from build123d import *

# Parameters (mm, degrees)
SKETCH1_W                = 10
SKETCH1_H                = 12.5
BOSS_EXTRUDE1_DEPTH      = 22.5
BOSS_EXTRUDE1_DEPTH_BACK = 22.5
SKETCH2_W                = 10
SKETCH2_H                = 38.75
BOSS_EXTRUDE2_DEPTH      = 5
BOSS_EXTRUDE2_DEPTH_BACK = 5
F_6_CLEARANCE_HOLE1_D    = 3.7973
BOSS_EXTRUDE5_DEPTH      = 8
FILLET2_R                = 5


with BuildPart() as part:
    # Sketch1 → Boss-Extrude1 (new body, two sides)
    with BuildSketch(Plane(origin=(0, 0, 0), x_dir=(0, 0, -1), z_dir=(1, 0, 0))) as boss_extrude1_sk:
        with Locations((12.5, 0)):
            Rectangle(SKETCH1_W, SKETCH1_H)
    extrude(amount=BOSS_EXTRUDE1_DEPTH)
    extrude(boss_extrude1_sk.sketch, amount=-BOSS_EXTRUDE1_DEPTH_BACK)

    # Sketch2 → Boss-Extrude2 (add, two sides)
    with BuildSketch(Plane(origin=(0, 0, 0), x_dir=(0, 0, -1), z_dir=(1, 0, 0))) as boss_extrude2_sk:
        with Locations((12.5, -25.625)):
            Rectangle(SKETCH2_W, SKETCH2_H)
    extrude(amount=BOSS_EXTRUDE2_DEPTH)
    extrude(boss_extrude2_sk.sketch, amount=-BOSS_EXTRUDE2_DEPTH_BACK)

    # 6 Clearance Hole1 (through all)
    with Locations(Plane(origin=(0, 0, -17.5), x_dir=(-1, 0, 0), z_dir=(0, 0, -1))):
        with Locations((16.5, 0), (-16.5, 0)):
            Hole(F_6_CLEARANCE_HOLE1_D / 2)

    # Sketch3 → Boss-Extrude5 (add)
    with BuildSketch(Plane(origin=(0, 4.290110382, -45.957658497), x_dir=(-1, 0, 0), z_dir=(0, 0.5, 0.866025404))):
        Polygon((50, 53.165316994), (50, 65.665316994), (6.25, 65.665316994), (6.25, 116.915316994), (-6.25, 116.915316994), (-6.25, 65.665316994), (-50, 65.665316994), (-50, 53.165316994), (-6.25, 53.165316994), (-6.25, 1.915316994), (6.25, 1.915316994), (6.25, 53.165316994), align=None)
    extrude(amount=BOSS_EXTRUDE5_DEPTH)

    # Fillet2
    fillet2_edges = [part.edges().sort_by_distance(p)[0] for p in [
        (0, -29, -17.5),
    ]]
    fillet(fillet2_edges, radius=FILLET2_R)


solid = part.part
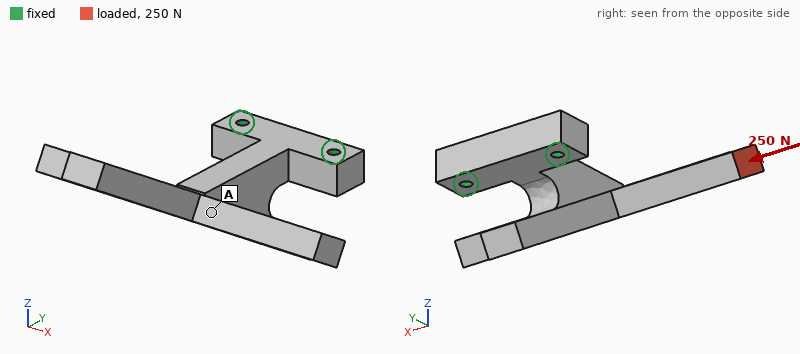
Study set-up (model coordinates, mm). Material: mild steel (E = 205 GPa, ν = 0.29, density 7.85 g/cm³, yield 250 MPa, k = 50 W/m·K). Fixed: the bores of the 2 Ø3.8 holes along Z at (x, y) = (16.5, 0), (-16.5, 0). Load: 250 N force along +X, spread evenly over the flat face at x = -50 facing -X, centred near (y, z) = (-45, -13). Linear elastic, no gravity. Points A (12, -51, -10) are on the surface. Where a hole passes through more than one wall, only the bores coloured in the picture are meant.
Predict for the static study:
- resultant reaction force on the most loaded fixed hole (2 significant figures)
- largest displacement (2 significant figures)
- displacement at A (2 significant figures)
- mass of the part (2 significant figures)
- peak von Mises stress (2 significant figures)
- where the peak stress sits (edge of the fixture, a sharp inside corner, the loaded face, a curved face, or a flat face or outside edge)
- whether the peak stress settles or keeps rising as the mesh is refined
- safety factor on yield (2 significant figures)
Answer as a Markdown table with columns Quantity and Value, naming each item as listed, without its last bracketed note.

| Quantity | Value |
|---|---|
| resultant reaction force on the most loaded fixed hole | 420 N |
| largest displacement | 91 µm |
| displacement at A | 42 µm |
| mass of the part | 230 g |
| peak von Mises stress | 65 MPa |
| where the peak stress sits | a curved face |
| whether the peak stress settles or keeps rising as the mesh is refined | settles |
| safety factor on yield | 3.8 |
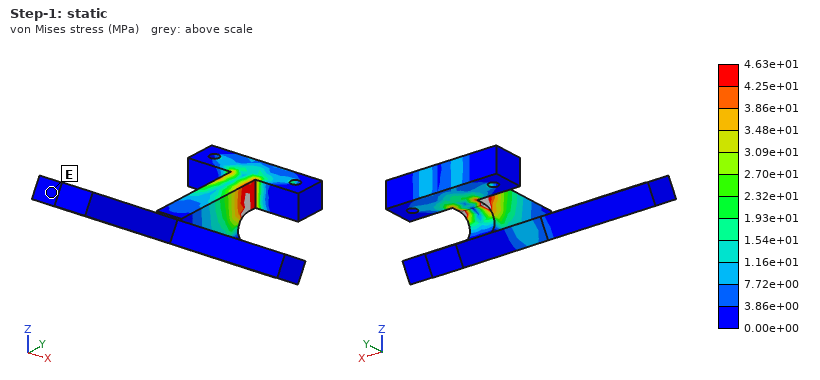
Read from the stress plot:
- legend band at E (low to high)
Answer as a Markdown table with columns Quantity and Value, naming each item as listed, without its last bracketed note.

| Quantity | Value |
|---|---|
| legend band at E | 0.00e+00 to 3.86e+00 MPa |
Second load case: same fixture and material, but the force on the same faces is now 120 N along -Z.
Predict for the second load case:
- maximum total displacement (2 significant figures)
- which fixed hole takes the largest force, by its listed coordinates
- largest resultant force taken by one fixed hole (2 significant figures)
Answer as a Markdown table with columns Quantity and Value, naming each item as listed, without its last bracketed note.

| Quantity | Value |
|---|---|
| maximum total displacement | 0.12 mm |
| which fixed hole takes the largest force, by its listed coordinates | (-16.5, 0) |
| largest resultant force taken by one fixed hole | 290 N |
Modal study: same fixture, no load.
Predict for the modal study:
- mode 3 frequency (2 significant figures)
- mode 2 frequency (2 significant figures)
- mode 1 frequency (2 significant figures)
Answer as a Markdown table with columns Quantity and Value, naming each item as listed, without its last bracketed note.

| Quantity | Value |
|---|---|
| mode 3 frequency | 1200 Hz |
| mode 2 frequency | 740 Hz |
| mode 1 frequency | 720 Hz |
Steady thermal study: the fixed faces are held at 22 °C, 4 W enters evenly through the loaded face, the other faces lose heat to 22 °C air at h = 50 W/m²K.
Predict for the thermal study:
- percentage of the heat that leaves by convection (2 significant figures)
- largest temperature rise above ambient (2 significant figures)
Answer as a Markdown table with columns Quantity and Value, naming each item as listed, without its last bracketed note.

| Quantity | Value |
|---|---|
| percentage of the heat that leaves by convection | 82 % |
| largest temperature rise above ambient | 33 K |
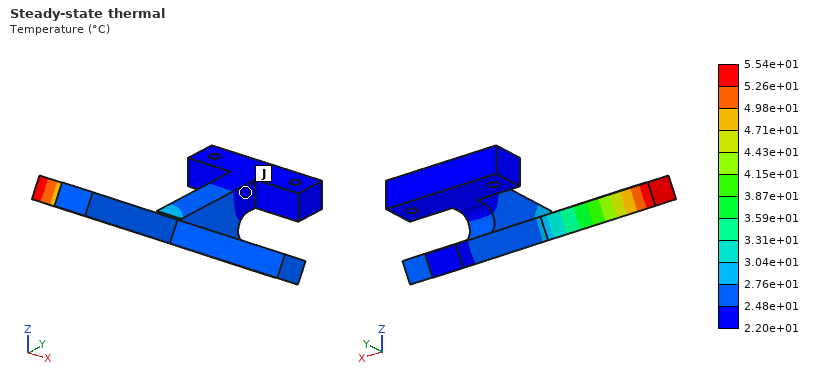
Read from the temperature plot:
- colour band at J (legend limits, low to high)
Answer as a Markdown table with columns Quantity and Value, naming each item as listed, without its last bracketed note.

| Quantity | Value |
|---|---|
| colour band at J | 2.20e+01 to 2.48e+01 °C |
